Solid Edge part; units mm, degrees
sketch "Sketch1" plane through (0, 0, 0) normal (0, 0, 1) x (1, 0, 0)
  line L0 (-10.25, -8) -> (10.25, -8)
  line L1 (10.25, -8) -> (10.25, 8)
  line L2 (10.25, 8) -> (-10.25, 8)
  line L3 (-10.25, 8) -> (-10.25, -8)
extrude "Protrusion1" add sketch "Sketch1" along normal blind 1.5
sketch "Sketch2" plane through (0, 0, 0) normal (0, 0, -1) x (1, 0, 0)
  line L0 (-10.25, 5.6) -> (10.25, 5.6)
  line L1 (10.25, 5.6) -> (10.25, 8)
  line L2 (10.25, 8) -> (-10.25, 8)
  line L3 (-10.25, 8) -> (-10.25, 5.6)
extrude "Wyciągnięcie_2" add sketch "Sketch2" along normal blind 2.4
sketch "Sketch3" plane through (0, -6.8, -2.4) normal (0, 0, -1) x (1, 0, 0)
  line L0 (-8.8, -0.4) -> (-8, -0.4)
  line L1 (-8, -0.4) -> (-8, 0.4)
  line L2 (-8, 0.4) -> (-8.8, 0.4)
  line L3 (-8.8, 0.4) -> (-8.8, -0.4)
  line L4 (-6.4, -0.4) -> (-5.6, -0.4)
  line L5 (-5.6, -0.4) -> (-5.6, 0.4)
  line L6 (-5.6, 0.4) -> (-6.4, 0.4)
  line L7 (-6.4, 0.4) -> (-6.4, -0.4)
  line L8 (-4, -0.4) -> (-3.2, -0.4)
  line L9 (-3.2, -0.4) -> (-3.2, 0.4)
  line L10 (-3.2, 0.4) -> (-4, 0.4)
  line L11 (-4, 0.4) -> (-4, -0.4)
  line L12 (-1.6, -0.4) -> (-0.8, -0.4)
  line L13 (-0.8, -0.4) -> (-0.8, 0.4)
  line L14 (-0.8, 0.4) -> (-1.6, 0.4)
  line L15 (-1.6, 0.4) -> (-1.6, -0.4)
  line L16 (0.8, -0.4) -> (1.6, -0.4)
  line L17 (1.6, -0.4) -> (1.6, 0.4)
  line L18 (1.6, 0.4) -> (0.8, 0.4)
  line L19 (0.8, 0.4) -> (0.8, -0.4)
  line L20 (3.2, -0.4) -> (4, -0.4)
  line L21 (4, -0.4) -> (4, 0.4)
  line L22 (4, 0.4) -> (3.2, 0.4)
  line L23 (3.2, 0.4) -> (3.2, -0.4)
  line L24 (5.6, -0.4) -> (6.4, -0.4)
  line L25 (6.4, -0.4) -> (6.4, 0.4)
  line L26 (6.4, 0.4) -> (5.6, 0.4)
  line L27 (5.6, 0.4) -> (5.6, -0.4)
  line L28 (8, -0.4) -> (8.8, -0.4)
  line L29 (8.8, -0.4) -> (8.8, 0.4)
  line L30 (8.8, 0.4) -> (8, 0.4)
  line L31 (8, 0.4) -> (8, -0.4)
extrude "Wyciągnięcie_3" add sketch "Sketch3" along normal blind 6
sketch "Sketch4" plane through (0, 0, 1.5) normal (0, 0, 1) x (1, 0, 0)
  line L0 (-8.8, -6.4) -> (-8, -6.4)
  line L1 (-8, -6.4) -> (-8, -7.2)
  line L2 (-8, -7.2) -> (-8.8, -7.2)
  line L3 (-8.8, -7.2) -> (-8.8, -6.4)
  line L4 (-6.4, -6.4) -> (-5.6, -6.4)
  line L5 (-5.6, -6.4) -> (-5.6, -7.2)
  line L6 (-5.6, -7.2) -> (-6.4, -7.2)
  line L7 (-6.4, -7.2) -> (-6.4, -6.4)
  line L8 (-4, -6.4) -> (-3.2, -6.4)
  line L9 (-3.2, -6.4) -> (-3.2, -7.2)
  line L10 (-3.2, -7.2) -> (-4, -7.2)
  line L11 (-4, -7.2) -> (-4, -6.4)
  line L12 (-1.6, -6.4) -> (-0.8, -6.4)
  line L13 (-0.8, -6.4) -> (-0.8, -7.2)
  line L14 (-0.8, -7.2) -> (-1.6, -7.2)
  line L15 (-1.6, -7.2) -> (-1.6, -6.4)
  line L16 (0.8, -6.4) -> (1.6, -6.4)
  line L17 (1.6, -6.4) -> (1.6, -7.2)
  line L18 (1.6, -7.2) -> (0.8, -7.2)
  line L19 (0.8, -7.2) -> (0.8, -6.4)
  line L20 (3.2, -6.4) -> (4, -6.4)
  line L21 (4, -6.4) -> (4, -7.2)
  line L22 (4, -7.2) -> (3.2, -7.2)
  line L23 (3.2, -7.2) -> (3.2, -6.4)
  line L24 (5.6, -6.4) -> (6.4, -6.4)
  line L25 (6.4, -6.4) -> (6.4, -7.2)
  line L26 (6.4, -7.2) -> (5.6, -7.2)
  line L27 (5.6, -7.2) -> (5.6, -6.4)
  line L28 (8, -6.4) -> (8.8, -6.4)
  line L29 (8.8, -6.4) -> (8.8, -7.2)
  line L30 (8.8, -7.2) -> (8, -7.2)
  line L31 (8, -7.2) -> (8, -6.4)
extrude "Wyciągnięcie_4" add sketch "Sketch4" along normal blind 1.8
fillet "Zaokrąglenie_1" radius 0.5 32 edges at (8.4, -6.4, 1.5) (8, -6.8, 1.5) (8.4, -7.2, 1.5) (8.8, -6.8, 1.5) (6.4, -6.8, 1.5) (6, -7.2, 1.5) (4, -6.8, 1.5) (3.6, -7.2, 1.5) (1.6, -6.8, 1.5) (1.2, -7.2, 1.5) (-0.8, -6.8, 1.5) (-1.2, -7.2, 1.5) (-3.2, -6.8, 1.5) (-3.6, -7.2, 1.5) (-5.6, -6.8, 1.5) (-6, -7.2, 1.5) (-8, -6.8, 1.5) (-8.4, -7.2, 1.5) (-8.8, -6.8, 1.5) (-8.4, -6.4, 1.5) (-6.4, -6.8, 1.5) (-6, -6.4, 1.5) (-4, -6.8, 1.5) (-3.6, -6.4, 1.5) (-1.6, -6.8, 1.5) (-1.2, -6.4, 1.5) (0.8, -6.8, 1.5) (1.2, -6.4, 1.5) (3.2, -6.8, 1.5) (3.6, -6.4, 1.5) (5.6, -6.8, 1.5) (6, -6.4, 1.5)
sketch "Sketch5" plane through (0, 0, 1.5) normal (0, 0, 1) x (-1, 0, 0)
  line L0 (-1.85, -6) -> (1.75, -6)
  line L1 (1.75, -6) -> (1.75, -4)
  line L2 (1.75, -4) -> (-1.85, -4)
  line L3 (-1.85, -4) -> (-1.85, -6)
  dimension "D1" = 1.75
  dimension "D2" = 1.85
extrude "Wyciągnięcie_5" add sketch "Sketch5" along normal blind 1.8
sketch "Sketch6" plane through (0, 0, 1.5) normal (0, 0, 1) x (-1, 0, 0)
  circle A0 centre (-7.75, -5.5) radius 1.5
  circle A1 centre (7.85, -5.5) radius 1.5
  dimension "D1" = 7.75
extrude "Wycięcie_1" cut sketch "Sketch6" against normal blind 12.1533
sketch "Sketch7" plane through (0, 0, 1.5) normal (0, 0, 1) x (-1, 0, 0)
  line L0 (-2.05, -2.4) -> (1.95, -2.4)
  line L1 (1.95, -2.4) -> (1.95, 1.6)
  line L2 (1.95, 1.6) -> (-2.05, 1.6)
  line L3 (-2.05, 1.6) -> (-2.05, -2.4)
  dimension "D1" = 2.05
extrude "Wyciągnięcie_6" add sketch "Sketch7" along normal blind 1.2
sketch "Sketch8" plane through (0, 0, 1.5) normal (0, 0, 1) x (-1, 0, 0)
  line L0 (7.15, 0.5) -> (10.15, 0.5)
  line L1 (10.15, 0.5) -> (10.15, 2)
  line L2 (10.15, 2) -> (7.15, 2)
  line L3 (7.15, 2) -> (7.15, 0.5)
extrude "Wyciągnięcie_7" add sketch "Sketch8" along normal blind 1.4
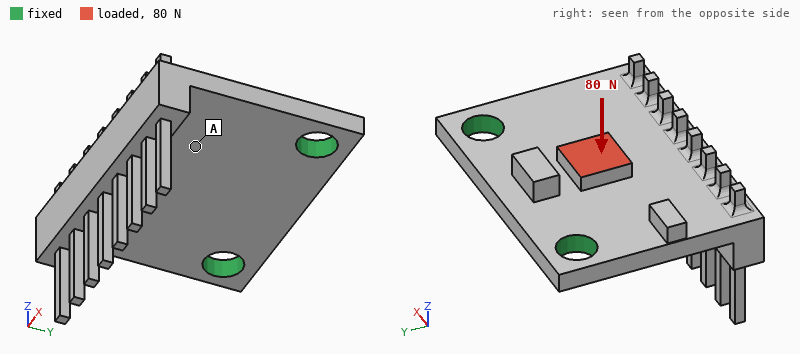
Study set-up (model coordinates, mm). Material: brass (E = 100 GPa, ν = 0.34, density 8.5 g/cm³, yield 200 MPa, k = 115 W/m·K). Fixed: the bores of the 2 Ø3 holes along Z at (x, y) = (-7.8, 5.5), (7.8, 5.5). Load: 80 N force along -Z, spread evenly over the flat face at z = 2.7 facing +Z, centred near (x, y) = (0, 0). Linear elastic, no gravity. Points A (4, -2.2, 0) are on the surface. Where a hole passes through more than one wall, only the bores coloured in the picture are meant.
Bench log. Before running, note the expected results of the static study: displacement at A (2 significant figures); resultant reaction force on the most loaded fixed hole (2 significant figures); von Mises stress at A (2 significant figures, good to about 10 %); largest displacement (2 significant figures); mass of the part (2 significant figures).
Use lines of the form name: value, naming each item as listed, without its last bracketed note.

displacement at A: 12 µm
resultant reaction force on the most loaded fixed hole: 42 N
von Mises stress at A: 11 MPa
largest displacement: 27 µm
mass of the part: 5.7 g
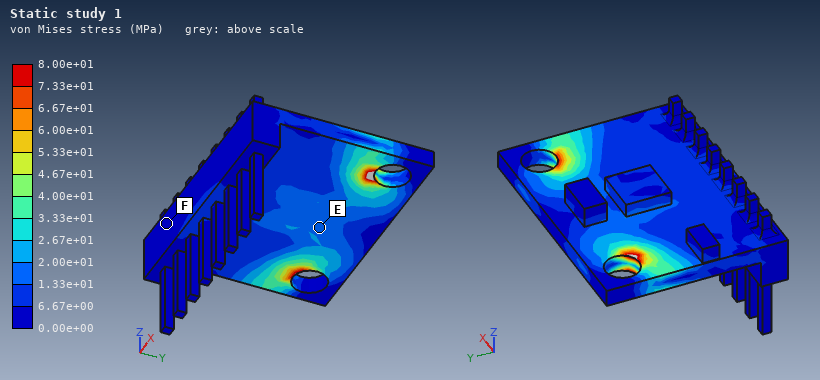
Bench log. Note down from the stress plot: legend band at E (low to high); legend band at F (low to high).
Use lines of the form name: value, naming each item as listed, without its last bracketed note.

legend band at E: 1.33e+01 to 2.00e+01 MPa
legend band at F: 0.00e+00 to 6.67e+00 MPa
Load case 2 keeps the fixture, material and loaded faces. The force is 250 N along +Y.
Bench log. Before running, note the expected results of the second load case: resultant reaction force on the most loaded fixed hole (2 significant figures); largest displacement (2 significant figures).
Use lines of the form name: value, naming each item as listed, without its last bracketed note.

resultant reaction force on the most loaded fixed hole: 140 N
largest displacement: 48 µm
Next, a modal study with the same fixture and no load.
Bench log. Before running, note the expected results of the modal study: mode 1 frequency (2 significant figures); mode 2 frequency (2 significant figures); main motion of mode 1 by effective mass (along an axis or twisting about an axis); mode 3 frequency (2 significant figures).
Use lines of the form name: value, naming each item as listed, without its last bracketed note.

mode 1 frequency: 3200 Hz
mode 2 frequency: 6800 Hz
main motion of mode 1 by effective mass: along Z
mode 3 frequency: 10 kHz
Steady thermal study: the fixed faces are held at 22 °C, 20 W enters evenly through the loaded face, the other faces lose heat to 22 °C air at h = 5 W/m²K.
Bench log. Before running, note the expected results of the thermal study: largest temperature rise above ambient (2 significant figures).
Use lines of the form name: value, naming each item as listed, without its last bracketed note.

largest temperature rise above ambient: 66 K
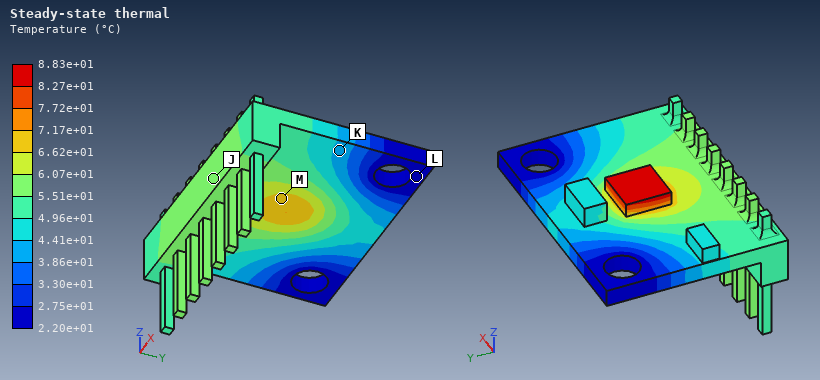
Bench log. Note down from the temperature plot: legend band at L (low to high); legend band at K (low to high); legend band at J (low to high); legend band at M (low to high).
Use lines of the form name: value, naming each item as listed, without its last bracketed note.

legend band at L: 2.20e+01 to 2.75e+01 °C
legend band at K: 3.86e+01 to 4.41e+01 °C
legend band at J: 5.51e+01 to 6.07e+01 °C
legend band at M: 6.62e+01 to 7.17e+01 °C
